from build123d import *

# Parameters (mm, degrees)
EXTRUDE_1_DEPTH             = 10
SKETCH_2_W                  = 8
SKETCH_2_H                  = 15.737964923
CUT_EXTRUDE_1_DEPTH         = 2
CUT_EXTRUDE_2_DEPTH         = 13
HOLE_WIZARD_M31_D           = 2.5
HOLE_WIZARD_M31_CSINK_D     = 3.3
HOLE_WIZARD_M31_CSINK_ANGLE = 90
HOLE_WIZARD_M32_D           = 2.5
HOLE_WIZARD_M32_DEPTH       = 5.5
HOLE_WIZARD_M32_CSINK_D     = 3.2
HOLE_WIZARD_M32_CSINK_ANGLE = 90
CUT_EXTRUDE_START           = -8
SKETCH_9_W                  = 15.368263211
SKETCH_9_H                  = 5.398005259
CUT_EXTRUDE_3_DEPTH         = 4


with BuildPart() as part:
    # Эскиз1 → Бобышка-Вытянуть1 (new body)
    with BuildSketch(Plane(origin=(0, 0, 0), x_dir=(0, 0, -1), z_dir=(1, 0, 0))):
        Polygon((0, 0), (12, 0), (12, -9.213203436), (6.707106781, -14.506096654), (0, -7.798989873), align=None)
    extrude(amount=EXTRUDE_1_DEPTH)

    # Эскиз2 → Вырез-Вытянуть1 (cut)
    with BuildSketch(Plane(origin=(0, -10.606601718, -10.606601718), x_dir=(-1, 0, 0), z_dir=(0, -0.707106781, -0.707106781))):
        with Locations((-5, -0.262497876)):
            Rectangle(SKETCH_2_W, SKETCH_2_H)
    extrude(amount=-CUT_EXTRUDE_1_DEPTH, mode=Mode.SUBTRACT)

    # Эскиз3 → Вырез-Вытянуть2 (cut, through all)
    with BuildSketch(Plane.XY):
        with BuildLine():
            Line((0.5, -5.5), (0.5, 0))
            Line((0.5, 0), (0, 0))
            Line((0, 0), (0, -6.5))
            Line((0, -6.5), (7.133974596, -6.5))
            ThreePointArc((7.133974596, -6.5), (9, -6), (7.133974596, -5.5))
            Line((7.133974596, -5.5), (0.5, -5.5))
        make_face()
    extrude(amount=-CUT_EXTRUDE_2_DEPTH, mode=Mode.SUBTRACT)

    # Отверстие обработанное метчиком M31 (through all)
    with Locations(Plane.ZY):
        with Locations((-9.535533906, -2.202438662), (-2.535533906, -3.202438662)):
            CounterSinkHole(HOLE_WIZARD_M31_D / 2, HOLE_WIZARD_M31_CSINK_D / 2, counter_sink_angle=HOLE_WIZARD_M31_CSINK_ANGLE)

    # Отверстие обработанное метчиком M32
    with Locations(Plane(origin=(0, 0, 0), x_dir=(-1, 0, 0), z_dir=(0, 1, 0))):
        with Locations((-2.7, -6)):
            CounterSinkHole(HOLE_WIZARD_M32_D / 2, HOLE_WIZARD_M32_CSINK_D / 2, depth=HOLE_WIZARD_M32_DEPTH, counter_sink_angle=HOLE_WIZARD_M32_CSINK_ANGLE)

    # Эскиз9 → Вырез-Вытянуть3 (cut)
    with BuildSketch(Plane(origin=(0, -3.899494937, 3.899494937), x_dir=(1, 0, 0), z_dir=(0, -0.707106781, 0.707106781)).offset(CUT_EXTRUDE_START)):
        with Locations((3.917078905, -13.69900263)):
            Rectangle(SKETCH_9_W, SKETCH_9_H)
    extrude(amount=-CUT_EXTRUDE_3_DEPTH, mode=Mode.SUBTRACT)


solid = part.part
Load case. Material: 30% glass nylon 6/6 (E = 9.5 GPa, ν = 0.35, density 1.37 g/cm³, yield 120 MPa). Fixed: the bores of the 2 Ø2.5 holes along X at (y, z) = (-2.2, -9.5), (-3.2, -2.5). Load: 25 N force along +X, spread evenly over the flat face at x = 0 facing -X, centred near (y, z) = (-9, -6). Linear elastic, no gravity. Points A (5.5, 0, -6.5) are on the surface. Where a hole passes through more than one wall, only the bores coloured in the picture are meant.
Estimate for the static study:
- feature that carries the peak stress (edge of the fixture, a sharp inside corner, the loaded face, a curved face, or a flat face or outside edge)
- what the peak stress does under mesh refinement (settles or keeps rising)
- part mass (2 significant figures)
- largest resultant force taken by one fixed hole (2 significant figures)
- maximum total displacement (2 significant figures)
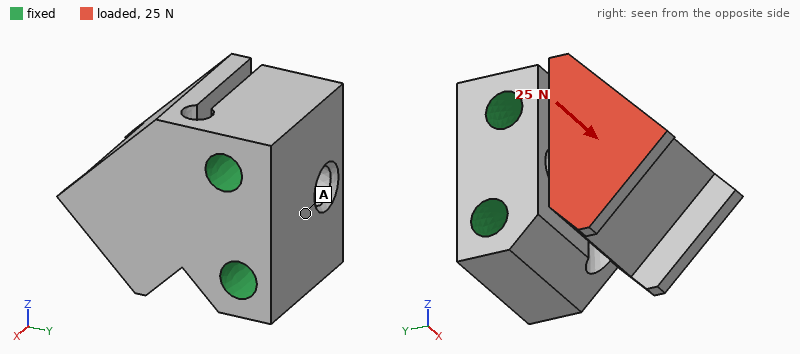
a sharp inside corner
keeps rising
1.3 g
13 N
0.26 mm
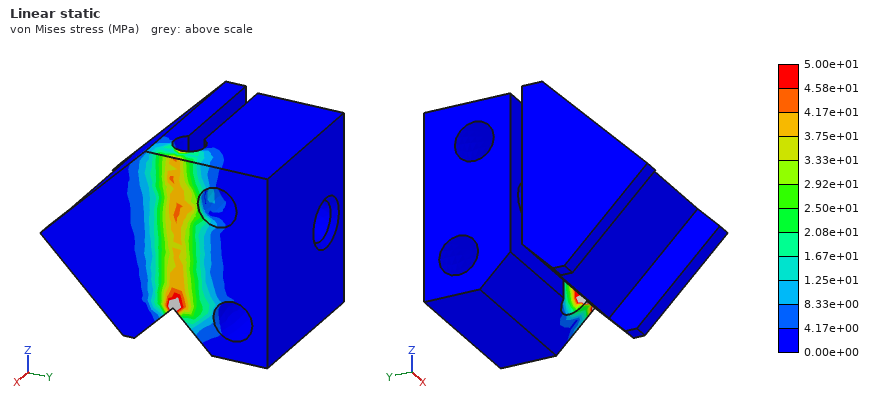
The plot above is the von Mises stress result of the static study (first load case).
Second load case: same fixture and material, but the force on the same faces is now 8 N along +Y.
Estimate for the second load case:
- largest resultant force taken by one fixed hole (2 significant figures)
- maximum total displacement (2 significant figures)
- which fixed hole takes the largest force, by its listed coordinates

4.9 N
0.22 mm
(-2.2, -9.5)
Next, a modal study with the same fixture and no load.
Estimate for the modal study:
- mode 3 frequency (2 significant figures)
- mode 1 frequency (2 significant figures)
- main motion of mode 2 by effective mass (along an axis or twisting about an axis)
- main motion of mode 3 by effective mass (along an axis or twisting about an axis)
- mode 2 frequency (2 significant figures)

15 kHz
2100 Hz
along Z
along X
6300 Hz
